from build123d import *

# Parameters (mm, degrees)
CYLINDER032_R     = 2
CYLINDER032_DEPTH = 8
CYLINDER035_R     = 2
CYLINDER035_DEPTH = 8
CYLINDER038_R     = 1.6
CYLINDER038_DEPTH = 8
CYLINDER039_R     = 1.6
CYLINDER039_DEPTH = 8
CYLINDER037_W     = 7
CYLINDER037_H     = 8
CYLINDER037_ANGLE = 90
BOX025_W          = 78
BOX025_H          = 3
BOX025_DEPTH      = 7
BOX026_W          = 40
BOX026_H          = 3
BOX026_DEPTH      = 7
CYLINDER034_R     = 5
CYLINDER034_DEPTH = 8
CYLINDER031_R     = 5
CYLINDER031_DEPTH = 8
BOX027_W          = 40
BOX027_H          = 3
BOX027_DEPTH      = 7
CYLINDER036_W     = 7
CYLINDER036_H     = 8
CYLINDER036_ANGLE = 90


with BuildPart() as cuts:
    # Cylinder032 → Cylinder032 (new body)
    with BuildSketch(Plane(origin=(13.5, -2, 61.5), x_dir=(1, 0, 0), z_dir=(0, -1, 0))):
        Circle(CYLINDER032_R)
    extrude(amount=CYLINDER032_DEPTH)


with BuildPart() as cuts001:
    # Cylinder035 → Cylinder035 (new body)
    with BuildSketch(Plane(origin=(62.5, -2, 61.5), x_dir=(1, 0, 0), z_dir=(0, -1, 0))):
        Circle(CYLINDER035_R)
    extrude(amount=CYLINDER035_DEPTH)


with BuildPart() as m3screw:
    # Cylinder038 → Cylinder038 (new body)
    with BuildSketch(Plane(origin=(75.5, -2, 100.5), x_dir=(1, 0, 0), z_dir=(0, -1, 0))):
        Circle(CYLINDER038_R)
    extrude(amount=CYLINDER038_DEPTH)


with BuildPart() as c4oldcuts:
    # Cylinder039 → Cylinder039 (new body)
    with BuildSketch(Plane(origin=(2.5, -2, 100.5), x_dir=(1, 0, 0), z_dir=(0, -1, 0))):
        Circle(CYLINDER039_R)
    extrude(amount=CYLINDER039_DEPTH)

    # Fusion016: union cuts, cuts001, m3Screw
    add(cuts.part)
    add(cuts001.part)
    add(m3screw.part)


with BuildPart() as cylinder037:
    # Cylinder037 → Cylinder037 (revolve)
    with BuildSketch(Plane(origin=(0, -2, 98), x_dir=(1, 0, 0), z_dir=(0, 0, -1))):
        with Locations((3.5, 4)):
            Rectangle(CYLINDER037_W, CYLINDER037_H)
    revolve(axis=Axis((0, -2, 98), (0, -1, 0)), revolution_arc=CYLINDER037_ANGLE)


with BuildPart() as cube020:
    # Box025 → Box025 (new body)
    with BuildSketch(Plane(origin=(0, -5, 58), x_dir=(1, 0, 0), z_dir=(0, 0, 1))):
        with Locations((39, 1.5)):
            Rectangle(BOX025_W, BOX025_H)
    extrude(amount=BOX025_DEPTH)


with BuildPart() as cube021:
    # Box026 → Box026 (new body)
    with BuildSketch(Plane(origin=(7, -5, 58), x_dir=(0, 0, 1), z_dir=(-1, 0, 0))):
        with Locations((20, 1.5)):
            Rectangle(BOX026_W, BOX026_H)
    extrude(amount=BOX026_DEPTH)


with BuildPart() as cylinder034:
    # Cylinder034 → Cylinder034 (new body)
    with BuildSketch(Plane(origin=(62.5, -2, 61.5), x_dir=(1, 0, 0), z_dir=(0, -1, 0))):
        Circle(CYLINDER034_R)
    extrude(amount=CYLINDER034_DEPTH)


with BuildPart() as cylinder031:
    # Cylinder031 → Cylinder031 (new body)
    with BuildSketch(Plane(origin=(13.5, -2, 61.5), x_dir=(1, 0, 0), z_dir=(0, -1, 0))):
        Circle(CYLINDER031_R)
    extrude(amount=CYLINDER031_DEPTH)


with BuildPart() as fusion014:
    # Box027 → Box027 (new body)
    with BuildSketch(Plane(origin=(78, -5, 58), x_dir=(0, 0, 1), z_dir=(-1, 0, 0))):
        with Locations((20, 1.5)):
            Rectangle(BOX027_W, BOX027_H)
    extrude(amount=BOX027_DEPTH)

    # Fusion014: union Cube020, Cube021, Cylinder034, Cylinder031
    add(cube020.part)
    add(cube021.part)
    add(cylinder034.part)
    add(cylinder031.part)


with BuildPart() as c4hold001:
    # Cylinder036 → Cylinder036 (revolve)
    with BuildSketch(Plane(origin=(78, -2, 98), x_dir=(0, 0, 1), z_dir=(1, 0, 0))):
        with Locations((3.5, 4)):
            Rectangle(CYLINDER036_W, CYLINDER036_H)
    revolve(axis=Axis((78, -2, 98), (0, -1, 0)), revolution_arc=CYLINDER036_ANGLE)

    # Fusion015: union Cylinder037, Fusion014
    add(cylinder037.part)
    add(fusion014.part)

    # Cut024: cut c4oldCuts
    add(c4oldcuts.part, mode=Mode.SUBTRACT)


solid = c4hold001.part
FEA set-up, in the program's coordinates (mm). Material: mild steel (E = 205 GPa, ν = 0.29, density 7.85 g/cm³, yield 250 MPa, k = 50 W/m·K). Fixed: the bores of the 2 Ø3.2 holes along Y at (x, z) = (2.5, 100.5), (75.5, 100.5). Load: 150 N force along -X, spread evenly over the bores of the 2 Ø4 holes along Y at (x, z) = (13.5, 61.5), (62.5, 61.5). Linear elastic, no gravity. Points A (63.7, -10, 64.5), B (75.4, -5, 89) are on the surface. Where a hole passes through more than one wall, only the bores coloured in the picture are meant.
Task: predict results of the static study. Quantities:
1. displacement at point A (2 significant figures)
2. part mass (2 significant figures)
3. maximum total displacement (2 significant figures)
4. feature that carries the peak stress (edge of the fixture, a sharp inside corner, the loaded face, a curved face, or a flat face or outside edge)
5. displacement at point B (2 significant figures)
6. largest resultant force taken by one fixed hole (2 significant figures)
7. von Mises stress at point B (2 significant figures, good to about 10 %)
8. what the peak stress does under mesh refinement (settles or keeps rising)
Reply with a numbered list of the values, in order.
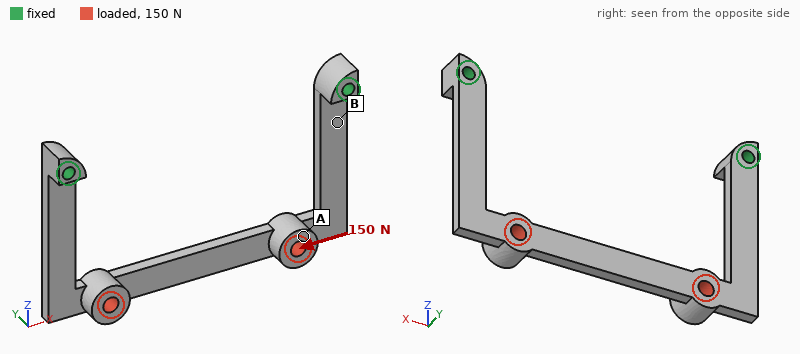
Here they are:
1. 38 µm
2. 33 g
3. 40 µm
4. edge of the fixture
5. 6.5 µm
6. 83 N
7. 13 MPa
8. keeps rising
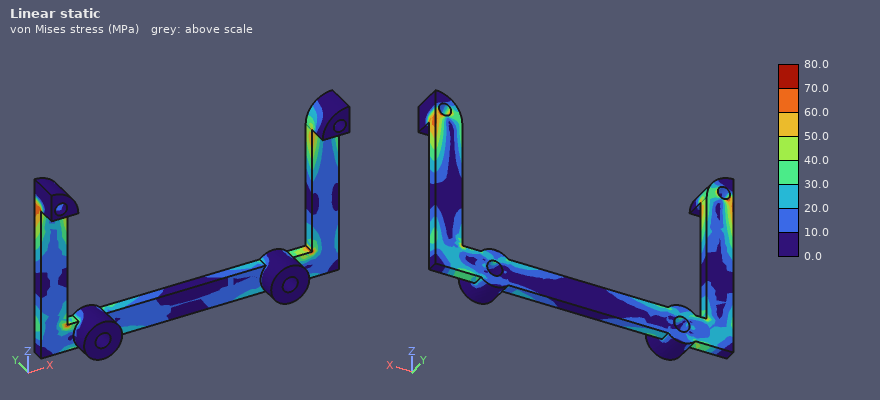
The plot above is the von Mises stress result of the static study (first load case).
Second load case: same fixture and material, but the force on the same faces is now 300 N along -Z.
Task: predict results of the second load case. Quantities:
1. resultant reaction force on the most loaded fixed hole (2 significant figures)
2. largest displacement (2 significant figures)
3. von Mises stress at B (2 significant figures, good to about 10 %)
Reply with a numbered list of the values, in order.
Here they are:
1. 160 N
2. 0.11 mm
3. 43 MPa
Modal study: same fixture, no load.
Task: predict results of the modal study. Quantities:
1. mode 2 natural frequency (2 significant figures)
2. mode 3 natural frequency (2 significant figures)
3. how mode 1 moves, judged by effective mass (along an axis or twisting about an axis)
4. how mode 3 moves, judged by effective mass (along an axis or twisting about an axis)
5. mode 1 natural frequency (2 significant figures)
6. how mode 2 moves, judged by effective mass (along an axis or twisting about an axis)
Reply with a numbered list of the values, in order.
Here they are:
1. 1400 Hz
2. 2300 Hz
3. along Y
4. along X
5. 640 Hz
6. twisting about Z
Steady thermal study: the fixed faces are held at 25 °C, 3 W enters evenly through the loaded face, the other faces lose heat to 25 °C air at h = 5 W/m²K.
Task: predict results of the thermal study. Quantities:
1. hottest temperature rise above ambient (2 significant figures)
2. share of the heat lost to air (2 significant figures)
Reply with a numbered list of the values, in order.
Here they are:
1. 53 K
2. 20 %
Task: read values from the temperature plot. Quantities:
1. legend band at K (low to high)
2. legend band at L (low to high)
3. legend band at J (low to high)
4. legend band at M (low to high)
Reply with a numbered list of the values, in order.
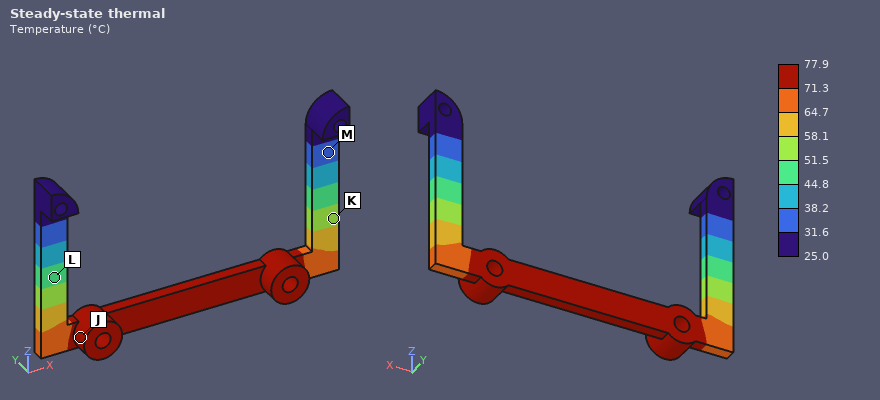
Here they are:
1. 51.5 to 58.1 °C
2. 44.8 to 51.5 °C
3. 71.3 to 77.9 °C
4. 31.6 to 38.2 °C
